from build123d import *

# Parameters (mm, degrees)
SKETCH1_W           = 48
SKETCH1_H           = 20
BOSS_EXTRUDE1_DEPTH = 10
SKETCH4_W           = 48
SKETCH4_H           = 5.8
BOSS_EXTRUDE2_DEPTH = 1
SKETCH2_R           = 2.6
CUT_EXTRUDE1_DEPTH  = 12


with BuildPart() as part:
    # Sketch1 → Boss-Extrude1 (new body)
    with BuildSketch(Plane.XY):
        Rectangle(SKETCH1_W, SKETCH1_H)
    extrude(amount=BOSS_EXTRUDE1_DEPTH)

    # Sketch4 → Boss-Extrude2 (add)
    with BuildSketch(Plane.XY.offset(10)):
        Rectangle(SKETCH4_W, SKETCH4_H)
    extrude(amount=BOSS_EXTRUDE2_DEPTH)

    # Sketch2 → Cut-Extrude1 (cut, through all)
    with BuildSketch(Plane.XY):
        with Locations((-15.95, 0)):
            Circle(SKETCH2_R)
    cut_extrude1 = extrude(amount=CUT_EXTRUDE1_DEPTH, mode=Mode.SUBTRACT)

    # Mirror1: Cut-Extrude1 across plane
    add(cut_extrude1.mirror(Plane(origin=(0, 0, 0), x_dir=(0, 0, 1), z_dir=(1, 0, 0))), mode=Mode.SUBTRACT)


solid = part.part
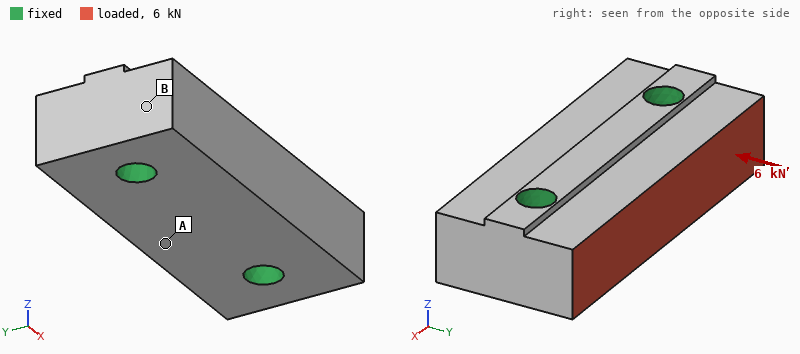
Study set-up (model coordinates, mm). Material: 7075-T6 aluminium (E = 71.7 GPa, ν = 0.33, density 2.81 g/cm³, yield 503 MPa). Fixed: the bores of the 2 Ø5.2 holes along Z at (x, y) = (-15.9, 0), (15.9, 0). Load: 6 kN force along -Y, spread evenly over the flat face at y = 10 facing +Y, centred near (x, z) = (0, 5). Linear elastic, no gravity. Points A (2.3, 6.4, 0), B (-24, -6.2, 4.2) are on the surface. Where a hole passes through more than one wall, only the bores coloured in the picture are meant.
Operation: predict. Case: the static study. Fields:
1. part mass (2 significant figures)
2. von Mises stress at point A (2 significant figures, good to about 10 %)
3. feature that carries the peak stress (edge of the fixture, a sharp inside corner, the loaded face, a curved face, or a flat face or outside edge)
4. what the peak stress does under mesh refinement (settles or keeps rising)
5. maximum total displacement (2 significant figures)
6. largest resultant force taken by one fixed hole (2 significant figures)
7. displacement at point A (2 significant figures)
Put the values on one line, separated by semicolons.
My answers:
26 g; 11 MPa; edge of the fixture; keeps rising; 5.4 µm; 3.0 kN; 4.9 µm
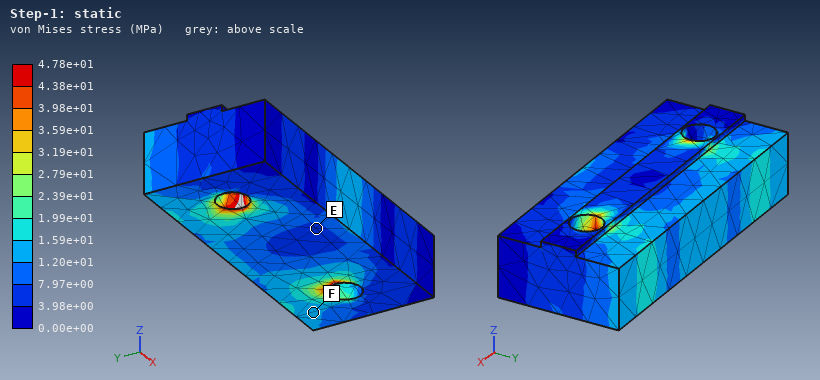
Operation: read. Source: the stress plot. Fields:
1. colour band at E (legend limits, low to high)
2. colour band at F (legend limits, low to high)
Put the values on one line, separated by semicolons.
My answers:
3.98e+00 to 7.97e+00 MPa; 1.20e+01 to 1.59e+01 MPa
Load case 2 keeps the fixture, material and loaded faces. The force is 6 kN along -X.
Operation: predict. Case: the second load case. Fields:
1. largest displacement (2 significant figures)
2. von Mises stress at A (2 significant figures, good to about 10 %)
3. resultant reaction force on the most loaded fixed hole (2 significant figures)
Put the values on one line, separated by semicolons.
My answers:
10 µm; 23 MPa; 3.3 kN
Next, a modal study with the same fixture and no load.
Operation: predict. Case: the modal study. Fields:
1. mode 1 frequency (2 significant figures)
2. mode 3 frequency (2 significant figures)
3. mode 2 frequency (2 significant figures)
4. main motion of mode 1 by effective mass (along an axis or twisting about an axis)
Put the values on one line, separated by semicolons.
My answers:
34 kHz; 37 kHz; 36 kHz; along Z
